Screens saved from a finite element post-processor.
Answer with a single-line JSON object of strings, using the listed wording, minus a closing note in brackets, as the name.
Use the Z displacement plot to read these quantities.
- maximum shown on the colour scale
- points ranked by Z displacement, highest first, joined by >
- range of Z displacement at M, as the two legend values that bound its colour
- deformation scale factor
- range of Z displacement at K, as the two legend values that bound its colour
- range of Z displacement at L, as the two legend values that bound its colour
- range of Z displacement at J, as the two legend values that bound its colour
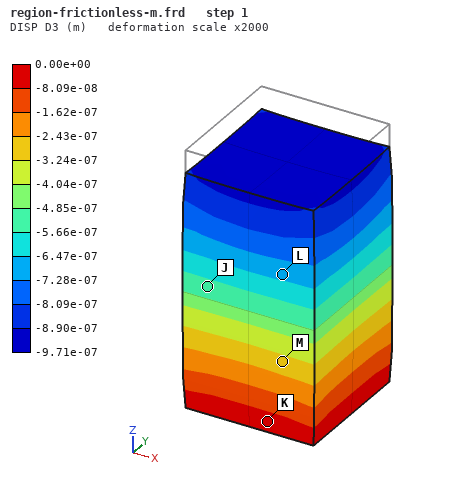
{"maximum shown on the colour scale": "0.00e+00 m", "points ranked by Z displacement, highest first, joined by >": "K > M > J > L", "range of Z displacement at M, as the two legend values that bound its colour": "-3.24e-07 to -2.43e-07 m", "deformation scale factor": "2000", "range of Z displacement at K, as the two legend values that bound its colour": "-8.09e-08 to 0.00e+00 m", "range of Z displacement at L, as the two legend values that bound its colour": "-7.28e-07 to -6.47e-07 m", "range of Z displacement at J, as the two legend values that bound its colour": "-5.66e-07 to -4.85e-07 m"}
